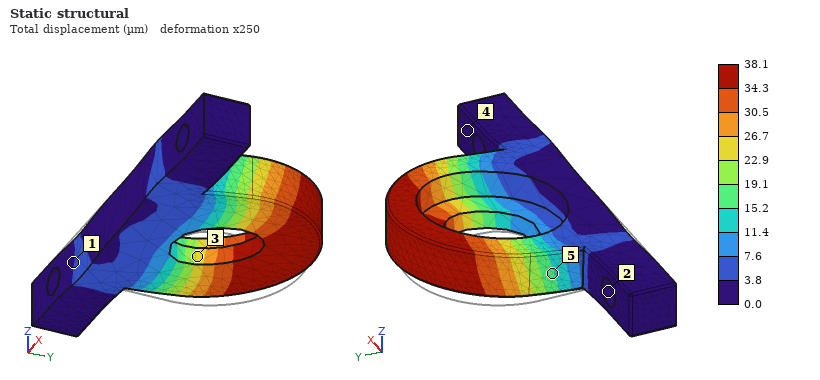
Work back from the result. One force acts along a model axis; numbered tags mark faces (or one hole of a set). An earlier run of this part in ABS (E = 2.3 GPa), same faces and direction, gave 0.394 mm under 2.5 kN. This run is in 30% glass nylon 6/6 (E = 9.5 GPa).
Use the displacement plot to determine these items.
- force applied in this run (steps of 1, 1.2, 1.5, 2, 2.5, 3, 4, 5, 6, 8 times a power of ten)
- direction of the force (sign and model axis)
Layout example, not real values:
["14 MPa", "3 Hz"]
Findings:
["1 kN", "+X"]
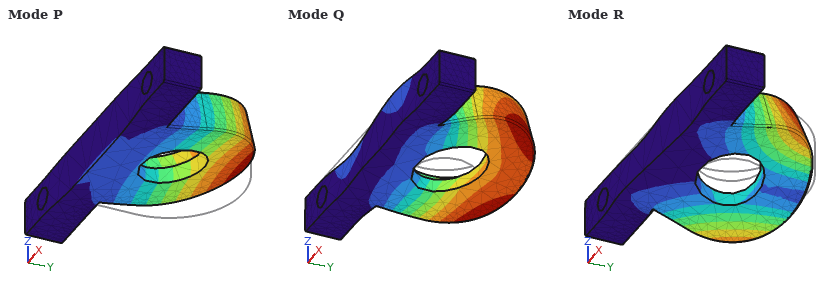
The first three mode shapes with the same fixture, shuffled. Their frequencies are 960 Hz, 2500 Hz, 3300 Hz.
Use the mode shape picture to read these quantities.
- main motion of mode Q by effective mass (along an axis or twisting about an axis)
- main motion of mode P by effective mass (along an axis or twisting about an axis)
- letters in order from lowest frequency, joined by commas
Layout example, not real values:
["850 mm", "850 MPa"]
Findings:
["along X", "along Z", "P, R, Q"]
